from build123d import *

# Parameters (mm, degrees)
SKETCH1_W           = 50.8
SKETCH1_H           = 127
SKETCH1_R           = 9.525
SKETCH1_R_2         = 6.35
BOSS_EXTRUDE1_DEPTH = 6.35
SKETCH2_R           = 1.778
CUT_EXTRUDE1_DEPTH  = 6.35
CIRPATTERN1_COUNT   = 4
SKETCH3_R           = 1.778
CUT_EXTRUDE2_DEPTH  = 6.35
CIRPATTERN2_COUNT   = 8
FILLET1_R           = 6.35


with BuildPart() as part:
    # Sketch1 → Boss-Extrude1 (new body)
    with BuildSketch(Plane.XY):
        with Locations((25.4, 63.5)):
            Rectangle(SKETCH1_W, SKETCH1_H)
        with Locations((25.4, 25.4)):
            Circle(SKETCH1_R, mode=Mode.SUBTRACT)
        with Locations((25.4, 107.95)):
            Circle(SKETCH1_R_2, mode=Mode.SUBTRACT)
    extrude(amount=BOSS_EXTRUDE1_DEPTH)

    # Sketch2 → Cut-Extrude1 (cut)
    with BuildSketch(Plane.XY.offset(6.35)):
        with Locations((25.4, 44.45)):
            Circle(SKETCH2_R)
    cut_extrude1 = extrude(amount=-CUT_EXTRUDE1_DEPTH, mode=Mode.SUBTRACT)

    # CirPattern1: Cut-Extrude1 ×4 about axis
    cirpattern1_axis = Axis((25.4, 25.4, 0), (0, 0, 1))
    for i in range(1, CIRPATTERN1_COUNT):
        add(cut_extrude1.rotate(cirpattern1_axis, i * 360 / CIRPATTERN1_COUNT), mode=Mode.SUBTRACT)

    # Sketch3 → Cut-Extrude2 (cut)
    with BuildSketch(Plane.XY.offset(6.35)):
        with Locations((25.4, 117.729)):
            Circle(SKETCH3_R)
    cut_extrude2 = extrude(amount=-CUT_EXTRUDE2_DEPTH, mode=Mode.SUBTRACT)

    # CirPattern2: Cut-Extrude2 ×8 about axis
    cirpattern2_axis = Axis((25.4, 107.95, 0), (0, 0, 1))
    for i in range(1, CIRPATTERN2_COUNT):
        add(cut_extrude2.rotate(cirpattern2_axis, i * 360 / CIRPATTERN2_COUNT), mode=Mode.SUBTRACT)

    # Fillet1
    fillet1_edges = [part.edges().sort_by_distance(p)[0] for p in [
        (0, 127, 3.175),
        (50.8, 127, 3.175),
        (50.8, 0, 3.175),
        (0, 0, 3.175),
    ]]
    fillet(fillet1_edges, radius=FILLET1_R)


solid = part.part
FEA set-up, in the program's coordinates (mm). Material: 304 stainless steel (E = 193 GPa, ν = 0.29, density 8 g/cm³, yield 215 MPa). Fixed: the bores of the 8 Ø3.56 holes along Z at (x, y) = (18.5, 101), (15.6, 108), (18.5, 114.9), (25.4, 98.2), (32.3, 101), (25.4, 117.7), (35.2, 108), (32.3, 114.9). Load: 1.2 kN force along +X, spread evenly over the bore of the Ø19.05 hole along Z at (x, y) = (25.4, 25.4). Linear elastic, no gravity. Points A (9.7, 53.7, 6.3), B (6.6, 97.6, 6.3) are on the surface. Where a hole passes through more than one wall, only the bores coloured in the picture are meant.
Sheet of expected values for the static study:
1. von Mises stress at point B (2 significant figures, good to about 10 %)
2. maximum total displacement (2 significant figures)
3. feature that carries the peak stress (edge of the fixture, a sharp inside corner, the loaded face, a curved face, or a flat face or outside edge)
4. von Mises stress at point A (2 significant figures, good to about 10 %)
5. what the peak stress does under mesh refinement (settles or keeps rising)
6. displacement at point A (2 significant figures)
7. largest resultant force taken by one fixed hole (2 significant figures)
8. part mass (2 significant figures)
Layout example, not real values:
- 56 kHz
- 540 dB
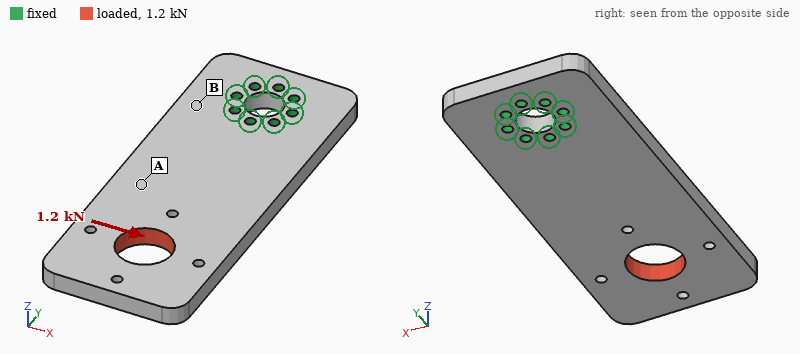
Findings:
- 21 MPa
- 39 µm
- edge of the fixture
- 9.0 MPa
- keeps rising
- 15 µm
- 1.5 kN
- 300 g
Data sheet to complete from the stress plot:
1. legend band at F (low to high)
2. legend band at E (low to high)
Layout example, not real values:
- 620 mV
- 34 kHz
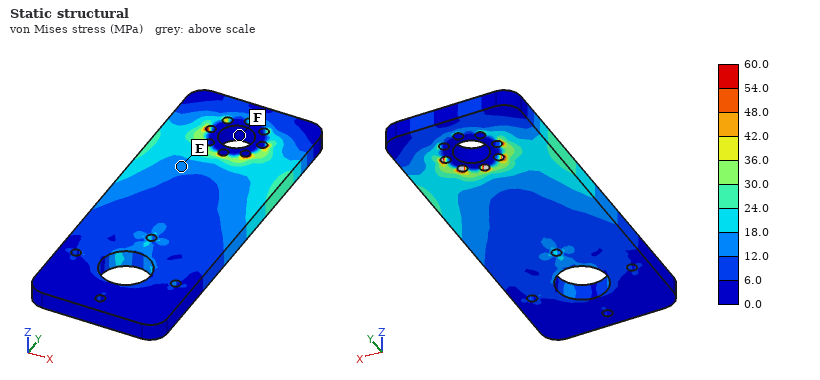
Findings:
- 0.0 to 6.0 MPa
- 12.0 to 18.0 MPa
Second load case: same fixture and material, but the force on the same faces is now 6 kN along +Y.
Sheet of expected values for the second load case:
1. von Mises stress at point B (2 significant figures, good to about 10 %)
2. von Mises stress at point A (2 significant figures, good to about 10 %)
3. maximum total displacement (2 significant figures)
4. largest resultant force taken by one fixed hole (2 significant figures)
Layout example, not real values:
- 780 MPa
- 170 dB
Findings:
- 12 MPa
- 19 MPa
- 11 µm
- 1.4 kN
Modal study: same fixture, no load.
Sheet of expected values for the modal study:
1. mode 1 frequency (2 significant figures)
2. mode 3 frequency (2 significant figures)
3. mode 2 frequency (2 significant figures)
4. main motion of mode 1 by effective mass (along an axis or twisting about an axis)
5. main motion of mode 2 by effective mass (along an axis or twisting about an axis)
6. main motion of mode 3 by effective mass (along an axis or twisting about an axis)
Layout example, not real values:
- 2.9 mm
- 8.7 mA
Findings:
- 540 Hz
- 2800 Hz
- 1900 Hz
- along Z
- twisting about Y
- along X
